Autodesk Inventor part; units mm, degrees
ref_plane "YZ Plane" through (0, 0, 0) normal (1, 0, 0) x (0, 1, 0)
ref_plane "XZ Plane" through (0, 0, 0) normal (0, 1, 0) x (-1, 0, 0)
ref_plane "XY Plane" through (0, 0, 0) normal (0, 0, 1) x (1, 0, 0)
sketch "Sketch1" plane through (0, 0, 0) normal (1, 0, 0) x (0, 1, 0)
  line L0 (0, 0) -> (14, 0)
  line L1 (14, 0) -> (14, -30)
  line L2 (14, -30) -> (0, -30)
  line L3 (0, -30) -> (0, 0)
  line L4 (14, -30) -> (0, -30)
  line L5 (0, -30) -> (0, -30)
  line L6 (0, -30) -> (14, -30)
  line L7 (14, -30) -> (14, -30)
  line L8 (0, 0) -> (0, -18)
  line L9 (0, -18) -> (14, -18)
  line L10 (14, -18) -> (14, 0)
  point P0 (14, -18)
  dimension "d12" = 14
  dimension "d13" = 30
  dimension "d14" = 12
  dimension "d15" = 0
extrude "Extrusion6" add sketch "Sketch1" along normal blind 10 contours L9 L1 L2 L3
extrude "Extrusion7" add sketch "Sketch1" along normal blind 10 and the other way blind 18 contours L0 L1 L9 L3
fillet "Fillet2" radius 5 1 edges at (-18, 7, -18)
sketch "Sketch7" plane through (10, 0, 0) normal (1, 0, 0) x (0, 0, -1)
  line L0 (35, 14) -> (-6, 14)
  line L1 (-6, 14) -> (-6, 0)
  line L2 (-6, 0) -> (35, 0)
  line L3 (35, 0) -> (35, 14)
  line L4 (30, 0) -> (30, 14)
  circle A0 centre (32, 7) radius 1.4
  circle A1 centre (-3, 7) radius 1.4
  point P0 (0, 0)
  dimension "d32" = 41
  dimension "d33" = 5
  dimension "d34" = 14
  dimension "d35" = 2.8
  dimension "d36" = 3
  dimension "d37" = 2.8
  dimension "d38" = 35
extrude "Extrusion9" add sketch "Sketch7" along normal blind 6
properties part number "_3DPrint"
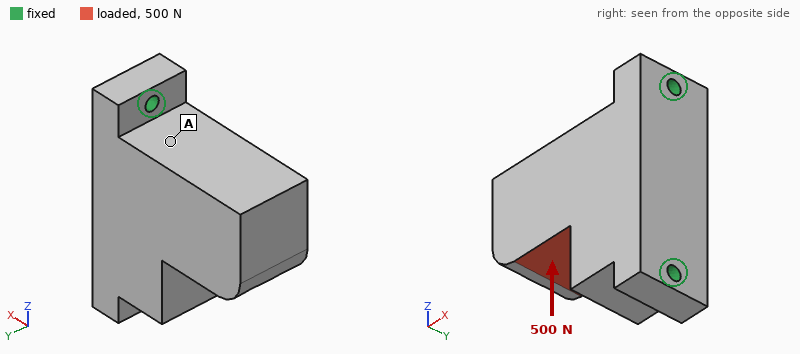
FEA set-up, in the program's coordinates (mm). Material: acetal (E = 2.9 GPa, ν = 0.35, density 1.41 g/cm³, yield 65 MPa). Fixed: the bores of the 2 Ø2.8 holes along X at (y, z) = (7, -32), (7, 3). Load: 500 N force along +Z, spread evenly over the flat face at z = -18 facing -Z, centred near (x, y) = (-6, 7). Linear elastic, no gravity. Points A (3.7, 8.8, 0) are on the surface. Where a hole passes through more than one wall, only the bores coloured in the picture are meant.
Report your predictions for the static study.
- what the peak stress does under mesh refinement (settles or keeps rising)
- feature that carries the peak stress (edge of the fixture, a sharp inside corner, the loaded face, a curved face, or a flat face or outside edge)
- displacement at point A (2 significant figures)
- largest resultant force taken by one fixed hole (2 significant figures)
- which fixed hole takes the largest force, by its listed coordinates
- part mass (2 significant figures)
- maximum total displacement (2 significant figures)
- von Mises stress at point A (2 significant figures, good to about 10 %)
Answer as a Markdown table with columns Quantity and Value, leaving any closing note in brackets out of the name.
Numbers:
| Quantity | Value |
|---|---|
| what the peak stress does under mesh refinement | keeps rising |
| feature that carries the peak stress | a sharp inside corner |
| displacement at point A | 0.052 mm |
| largest resultant force taken by one fixed hole | 420 N |
| which fixed hole takes the largest force, by its listed coordinates | (7, -32) |
| part mass | 17 g |
| maximum total displacement | 0.14 mm |
| von Mises stress at point A | 4.6 MPa |
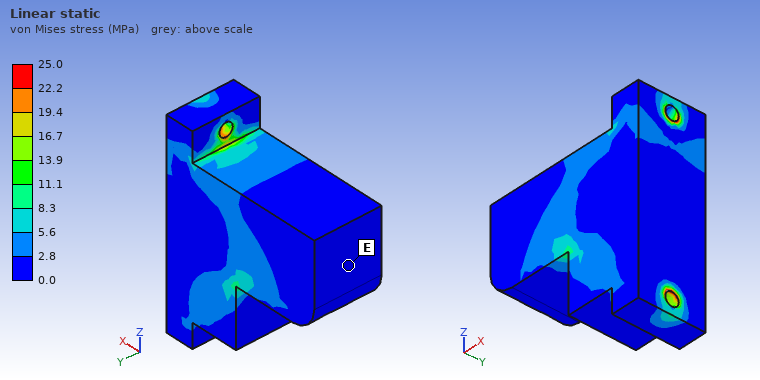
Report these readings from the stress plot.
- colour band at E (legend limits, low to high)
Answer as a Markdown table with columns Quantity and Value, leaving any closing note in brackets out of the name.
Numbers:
| Quantity | Value |
|---|---|
| colour band at E | 0.0 to 2.8 MPa |
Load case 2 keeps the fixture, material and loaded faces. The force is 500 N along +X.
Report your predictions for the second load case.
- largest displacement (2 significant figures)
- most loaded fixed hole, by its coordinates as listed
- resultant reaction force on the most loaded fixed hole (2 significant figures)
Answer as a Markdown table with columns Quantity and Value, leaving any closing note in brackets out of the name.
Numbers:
| Quantity | Value |
|---|---|
| largest displacement | 98 µm |
| most loaded fixed hole, by its coordinates as listed | (7, -32) |
| resultant reaction force on the most loaded fixed hole | 340 N |
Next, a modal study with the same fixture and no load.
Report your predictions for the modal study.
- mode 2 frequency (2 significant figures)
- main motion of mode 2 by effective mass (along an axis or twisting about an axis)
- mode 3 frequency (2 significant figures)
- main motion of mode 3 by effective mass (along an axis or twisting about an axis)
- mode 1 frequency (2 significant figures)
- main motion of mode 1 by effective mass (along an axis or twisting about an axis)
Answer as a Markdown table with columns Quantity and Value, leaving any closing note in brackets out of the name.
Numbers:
| Quantity | Value |
|---|---|
| mode 2 frequency | 3800 Hz |
| main motion of mode 2 by effective mass | along Z |
| mode 3 frequency | 4800 Hz |
| main motion of mode 3 by effective mass | along X |
| mode 1 frequency | 1300 Hz |
| main motion of mode 1 by effective mass | along Y |
